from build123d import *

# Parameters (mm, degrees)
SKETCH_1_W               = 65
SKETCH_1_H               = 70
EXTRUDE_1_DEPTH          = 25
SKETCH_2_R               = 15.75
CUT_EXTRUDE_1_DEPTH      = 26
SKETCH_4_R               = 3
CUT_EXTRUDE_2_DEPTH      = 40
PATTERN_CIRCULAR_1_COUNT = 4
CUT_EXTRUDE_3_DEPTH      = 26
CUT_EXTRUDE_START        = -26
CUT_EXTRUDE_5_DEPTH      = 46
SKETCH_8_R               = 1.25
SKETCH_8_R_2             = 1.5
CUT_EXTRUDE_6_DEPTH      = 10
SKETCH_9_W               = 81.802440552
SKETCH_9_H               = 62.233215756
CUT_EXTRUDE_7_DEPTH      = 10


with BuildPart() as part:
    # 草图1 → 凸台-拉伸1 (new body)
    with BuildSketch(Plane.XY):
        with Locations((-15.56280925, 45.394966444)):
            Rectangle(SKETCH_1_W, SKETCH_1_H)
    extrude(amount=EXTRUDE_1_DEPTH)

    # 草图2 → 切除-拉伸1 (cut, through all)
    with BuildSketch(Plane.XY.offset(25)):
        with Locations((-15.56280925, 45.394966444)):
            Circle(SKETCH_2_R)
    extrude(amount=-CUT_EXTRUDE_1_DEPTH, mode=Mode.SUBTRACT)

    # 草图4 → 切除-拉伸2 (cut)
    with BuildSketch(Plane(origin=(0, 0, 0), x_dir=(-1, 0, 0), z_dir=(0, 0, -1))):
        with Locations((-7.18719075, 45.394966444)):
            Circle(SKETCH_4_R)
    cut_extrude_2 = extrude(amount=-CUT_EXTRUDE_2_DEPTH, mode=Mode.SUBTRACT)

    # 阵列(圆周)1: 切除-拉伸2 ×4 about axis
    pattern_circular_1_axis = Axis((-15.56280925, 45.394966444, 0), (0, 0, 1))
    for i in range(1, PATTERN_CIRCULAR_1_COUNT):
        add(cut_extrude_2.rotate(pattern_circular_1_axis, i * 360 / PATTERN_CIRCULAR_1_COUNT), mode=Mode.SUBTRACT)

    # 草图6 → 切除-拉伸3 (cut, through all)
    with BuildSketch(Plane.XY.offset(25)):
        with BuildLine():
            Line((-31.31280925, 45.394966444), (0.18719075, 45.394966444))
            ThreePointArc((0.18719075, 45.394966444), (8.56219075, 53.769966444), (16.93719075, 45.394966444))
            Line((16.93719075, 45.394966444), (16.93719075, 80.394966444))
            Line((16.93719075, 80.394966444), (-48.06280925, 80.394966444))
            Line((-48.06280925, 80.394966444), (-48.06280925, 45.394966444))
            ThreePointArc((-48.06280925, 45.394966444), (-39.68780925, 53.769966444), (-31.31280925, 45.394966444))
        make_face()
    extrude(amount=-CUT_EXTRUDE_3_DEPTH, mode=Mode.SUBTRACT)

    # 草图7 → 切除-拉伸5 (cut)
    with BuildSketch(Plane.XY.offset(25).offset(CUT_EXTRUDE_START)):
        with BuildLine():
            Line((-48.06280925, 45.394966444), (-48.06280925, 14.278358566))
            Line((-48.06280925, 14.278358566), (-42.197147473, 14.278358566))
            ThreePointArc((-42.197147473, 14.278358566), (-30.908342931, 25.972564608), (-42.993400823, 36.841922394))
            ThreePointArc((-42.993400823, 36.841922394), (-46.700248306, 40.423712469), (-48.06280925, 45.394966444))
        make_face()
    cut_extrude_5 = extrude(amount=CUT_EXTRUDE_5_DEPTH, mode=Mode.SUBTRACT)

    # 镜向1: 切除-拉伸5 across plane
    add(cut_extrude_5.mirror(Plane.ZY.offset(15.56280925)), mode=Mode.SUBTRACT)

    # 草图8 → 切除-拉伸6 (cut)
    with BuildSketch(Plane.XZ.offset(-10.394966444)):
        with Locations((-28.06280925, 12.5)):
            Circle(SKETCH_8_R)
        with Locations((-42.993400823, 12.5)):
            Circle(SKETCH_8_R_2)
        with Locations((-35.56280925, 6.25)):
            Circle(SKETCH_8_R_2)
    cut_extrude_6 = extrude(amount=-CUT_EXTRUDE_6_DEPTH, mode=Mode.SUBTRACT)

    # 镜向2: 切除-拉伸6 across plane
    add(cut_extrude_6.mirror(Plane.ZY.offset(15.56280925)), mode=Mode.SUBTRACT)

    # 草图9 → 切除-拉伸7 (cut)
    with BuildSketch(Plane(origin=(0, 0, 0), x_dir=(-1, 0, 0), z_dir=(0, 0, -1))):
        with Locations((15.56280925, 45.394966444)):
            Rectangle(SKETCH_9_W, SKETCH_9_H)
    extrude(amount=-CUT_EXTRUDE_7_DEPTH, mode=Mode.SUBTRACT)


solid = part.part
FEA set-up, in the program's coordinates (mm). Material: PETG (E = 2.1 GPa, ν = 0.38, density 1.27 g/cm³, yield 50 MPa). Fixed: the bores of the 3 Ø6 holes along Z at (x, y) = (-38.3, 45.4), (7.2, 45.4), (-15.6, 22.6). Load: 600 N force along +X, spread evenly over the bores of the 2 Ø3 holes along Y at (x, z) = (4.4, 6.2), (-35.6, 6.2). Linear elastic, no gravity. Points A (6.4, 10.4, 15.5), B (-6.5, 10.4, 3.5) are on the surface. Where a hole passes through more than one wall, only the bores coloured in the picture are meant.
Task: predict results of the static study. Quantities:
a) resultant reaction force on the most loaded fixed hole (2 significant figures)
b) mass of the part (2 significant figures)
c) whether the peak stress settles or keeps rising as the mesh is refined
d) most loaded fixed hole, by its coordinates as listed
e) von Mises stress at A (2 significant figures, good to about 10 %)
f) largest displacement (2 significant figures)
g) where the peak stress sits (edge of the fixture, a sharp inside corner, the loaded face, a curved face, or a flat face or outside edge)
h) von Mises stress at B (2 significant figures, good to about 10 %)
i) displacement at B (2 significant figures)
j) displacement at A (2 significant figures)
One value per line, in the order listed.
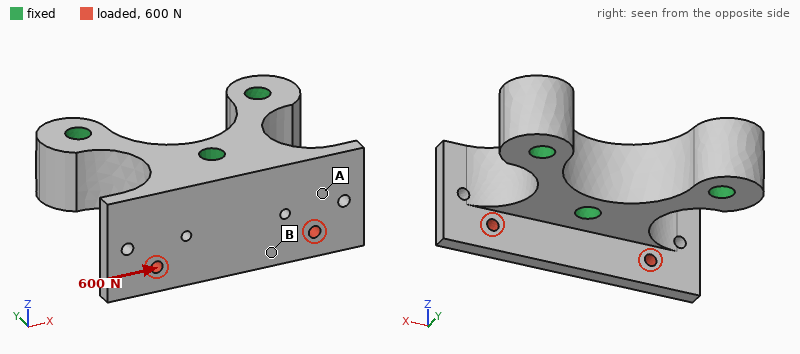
550 N
28 g
keeps rising
(-15.6, 22.6)
1.9 MPa
0.27 mm
edge of the fixture
4.4 MPa
0.13 mm
0.13 mm
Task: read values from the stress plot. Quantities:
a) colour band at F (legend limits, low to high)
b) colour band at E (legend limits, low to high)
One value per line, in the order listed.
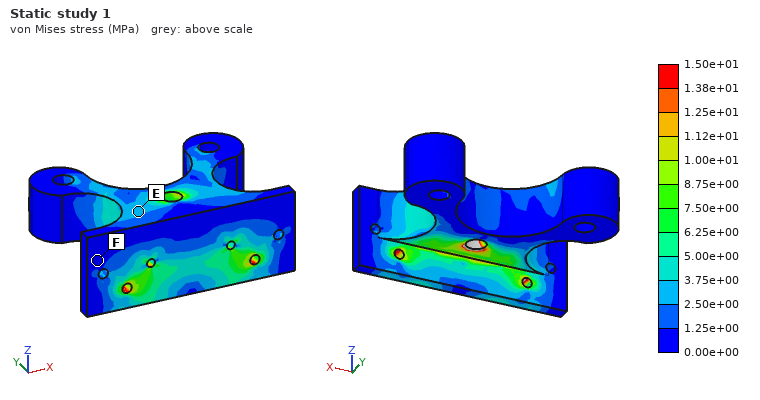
0.00e+00 to 1.25e+00 MPa
2.50e+00 to 3.75e+00 MPa
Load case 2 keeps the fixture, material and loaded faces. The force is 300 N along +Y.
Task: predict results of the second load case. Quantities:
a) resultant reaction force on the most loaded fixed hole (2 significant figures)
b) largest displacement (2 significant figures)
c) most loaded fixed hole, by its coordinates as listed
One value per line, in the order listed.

190 N
0.36 mm
(-15.6, 22.6)
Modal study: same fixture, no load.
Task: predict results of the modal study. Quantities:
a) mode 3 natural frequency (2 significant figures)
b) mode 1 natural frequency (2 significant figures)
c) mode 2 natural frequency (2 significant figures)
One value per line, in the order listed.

3000 Hz
2600 Hz
2900 Hz
